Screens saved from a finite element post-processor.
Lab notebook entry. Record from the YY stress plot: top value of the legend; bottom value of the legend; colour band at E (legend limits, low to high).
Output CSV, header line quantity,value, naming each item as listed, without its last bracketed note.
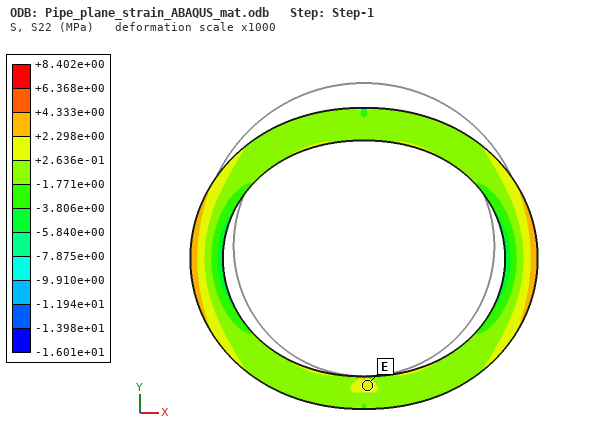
quantity,value
top value of the legend,+8.402e+00 MPa
bottom value of the legend,-1.601e+01 MPa
colour band at E,+2.636e-01 to +2.298e+00 MPa
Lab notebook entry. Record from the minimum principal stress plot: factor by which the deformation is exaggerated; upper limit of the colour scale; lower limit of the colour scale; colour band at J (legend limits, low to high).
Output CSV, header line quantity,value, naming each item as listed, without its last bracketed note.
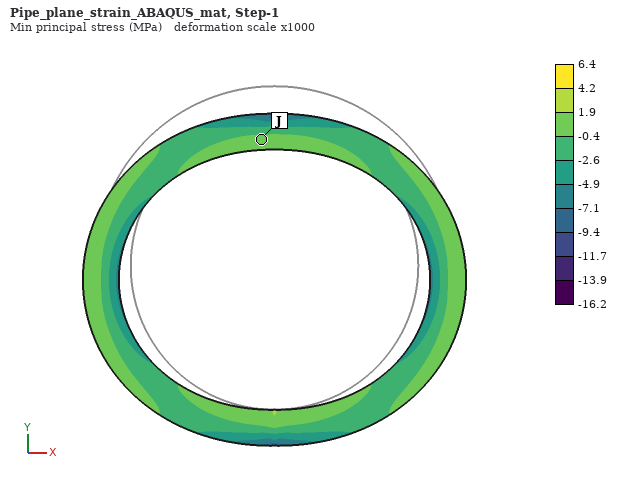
quantity,value
factor by which the deformation is exaggerated,1000
upper limit of the colour scale,6.4 MPa
lower limit of the colour scale,-16.2 MPa
colour band at J,-0.4 to 1.9 MPa
